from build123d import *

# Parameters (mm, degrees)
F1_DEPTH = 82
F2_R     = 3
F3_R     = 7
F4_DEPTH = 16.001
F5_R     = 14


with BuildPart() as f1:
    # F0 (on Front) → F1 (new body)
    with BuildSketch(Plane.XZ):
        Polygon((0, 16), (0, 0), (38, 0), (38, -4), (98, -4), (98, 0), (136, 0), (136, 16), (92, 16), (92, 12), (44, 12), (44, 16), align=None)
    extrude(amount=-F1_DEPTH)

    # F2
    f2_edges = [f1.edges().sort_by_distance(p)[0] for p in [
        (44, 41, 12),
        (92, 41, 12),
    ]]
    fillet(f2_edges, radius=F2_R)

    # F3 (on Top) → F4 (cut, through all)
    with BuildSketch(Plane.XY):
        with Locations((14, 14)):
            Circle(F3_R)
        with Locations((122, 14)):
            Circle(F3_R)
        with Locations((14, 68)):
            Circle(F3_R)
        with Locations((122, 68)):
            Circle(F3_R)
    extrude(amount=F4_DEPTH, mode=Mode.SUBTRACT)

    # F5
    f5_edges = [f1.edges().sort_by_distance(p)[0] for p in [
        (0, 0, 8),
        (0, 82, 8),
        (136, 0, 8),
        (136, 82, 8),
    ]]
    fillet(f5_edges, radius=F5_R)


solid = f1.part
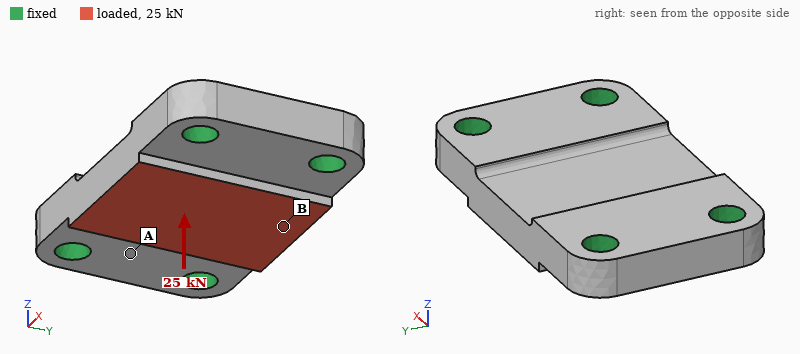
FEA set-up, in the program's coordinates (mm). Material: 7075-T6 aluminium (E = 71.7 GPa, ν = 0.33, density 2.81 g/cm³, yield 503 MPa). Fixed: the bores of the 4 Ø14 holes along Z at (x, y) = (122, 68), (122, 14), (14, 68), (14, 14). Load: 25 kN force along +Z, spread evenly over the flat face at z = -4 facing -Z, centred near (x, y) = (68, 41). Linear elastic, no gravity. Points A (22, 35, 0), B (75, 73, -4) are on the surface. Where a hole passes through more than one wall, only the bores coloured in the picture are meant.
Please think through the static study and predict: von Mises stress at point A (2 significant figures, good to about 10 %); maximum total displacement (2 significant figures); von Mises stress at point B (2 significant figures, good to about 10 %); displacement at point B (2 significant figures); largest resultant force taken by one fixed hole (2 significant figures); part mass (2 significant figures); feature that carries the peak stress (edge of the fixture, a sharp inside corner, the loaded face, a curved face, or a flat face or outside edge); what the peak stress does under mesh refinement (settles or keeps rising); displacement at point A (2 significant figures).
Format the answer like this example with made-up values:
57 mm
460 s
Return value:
19 MPa
64 µm
47 MPa
59 µm
8.0 kN
480 g
edge of the fixture
keeps rising
11 µm
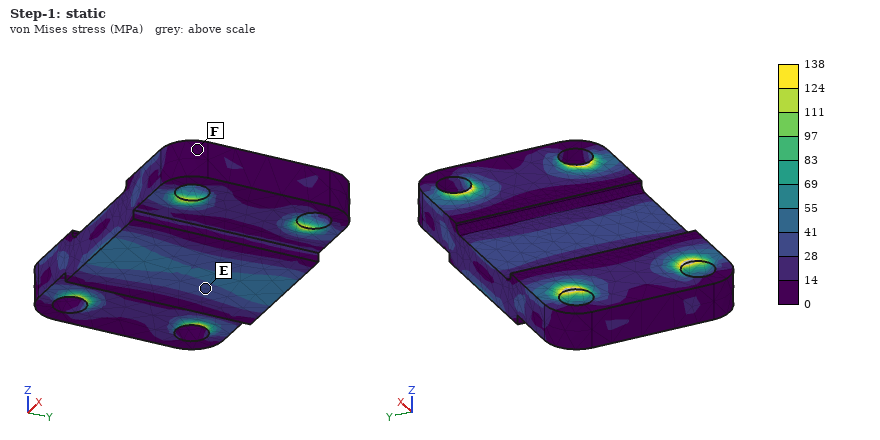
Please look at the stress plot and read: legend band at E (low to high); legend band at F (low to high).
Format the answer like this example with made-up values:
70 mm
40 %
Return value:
28 to 41 MPa
0 to 14 MPa
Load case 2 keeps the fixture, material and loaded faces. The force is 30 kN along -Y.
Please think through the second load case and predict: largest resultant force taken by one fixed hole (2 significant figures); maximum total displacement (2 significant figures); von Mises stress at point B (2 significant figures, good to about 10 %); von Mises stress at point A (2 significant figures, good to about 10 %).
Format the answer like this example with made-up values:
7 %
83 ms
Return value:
10 kN
51 µm
20 MPa
27 MPa
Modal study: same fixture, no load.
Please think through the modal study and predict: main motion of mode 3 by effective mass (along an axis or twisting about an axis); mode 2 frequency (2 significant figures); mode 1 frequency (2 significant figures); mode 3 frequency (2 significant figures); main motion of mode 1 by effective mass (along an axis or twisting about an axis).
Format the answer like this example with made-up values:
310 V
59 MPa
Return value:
along Y
8900 Hz
7000 Hz
13 kHz
along Z
